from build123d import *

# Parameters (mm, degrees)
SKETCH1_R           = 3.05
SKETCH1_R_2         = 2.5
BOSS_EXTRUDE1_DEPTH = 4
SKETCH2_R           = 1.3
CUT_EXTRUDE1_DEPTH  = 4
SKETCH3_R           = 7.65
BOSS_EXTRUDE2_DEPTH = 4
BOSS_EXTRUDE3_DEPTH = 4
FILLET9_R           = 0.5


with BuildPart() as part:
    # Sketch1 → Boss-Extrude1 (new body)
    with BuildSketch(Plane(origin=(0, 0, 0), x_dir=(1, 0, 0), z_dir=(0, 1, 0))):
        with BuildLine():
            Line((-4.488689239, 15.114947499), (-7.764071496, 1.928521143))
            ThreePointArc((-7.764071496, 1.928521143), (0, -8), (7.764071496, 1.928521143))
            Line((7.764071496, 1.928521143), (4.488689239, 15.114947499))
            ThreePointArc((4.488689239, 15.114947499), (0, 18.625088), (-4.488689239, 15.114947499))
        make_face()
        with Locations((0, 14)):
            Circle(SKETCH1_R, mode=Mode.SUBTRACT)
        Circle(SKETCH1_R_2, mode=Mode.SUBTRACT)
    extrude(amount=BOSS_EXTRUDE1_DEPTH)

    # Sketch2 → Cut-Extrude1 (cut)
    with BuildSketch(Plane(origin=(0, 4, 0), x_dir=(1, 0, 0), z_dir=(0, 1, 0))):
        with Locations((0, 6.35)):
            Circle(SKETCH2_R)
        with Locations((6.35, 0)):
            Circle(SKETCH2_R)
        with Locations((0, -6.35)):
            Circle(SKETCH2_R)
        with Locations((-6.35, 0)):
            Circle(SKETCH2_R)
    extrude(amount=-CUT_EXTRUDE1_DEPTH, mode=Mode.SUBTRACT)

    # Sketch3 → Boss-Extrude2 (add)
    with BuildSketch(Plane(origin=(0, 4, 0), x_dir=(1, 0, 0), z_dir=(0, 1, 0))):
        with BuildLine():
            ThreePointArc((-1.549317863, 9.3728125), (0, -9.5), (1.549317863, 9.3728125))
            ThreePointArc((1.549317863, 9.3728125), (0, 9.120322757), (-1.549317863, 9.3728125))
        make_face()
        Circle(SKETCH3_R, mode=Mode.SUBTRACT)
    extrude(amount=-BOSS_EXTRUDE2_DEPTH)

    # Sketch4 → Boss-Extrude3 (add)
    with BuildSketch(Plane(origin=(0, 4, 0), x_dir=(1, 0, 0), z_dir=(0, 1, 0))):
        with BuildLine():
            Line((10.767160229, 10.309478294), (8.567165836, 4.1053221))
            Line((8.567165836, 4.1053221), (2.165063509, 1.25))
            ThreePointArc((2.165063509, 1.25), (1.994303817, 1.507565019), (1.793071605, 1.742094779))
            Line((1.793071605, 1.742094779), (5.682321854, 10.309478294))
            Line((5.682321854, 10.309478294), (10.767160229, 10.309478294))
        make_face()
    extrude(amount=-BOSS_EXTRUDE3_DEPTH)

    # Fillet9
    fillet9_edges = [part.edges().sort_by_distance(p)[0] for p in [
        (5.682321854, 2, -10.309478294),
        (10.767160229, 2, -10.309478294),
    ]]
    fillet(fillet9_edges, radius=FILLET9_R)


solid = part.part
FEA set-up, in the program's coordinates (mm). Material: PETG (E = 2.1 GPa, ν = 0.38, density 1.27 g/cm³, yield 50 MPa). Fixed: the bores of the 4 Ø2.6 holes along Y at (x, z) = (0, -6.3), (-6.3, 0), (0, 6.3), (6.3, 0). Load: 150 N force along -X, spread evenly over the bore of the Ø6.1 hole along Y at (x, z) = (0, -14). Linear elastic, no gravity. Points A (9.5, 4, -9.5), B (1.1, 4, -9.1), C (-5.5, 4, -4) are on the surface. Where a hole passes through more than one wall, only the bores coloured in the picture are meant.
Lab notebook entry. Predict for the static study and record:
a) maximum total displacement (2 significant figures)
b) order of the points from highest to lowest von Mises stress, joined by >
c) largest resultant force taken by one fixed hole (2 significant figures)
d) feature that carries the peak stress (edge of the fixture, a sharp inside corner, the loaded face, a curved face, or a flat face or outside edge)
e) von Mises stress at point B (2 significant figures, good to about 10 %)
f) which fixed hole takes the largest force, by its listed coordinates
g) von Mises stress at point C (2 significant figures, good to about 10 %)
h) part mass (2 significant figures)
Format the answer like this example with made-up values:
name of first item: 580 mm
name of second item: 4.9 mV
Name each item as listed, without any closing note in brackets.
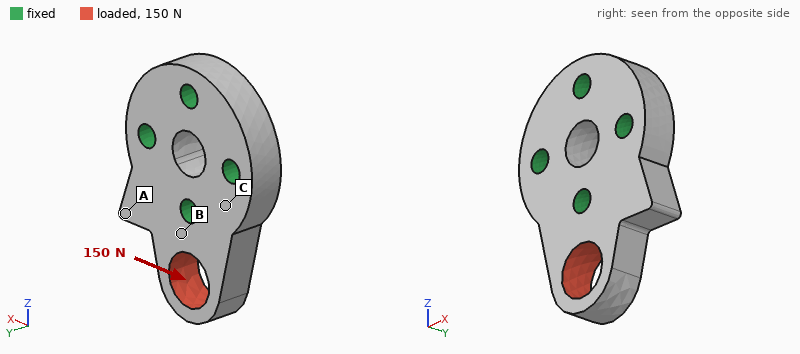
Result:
maximum total displacement: 0.21 mm
order of the points from highest to lowest von Mises stress, joined by >: B > C > A
largest resultant force taken by one fixed hole: 150 N
feature that carries the peak stress: a curved face
von Mises stress at point B: 10 MPa
which fixed hole takes the largest force, by its listed coordinates: (0, -6.3)
von Mises stress at point C: 5.1 MPa
part mass: 1.6 g
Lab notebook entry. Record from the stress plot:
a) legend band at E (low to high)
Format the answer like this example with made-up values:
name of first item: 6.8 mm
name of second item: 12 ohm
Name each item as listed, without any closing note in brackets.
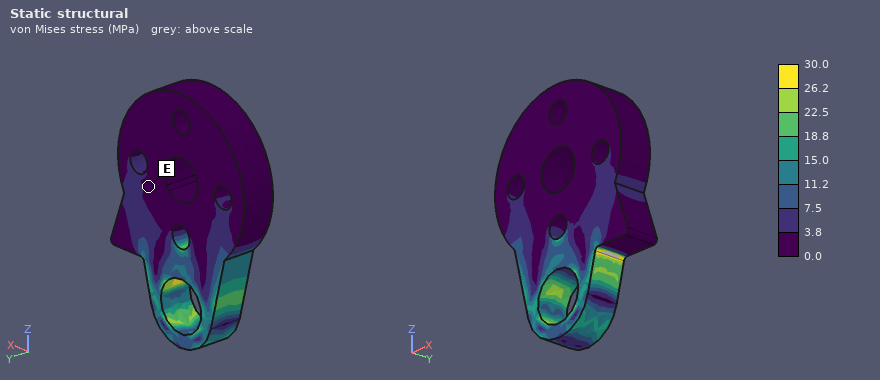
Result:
legend band at E: 0.0 to 3.8 MPa
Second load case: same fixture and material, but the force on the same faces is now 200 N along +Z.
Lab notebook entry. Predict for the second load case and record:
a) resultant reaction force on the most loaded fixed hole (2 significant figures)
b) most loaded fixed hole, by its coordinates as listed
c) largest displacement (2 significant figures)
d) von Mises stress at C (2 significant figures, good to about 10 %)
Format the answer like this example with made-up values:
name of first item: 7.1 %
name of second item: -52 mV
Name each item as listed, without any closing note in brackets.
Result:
resultant reaction force on the most loaded fixed hole: 110 N
most loaded fixed hole, by its coordinates as listed: (0, -6.3)
largest displacement: 69 µm
von Mises stress at C: 3.0 MPa
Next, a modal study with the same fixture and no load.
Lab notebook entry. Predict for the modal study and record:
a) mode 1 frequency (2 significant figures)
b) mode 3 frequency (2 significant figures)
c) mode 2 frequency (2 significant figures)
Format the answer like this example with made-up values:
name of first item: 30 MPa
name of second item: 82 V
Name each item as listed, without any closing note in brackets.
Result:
mode 1 frequency: 7100 Hz
mode 3 frequency: 11 kHz
mode 2 frequency: 11 kHz
